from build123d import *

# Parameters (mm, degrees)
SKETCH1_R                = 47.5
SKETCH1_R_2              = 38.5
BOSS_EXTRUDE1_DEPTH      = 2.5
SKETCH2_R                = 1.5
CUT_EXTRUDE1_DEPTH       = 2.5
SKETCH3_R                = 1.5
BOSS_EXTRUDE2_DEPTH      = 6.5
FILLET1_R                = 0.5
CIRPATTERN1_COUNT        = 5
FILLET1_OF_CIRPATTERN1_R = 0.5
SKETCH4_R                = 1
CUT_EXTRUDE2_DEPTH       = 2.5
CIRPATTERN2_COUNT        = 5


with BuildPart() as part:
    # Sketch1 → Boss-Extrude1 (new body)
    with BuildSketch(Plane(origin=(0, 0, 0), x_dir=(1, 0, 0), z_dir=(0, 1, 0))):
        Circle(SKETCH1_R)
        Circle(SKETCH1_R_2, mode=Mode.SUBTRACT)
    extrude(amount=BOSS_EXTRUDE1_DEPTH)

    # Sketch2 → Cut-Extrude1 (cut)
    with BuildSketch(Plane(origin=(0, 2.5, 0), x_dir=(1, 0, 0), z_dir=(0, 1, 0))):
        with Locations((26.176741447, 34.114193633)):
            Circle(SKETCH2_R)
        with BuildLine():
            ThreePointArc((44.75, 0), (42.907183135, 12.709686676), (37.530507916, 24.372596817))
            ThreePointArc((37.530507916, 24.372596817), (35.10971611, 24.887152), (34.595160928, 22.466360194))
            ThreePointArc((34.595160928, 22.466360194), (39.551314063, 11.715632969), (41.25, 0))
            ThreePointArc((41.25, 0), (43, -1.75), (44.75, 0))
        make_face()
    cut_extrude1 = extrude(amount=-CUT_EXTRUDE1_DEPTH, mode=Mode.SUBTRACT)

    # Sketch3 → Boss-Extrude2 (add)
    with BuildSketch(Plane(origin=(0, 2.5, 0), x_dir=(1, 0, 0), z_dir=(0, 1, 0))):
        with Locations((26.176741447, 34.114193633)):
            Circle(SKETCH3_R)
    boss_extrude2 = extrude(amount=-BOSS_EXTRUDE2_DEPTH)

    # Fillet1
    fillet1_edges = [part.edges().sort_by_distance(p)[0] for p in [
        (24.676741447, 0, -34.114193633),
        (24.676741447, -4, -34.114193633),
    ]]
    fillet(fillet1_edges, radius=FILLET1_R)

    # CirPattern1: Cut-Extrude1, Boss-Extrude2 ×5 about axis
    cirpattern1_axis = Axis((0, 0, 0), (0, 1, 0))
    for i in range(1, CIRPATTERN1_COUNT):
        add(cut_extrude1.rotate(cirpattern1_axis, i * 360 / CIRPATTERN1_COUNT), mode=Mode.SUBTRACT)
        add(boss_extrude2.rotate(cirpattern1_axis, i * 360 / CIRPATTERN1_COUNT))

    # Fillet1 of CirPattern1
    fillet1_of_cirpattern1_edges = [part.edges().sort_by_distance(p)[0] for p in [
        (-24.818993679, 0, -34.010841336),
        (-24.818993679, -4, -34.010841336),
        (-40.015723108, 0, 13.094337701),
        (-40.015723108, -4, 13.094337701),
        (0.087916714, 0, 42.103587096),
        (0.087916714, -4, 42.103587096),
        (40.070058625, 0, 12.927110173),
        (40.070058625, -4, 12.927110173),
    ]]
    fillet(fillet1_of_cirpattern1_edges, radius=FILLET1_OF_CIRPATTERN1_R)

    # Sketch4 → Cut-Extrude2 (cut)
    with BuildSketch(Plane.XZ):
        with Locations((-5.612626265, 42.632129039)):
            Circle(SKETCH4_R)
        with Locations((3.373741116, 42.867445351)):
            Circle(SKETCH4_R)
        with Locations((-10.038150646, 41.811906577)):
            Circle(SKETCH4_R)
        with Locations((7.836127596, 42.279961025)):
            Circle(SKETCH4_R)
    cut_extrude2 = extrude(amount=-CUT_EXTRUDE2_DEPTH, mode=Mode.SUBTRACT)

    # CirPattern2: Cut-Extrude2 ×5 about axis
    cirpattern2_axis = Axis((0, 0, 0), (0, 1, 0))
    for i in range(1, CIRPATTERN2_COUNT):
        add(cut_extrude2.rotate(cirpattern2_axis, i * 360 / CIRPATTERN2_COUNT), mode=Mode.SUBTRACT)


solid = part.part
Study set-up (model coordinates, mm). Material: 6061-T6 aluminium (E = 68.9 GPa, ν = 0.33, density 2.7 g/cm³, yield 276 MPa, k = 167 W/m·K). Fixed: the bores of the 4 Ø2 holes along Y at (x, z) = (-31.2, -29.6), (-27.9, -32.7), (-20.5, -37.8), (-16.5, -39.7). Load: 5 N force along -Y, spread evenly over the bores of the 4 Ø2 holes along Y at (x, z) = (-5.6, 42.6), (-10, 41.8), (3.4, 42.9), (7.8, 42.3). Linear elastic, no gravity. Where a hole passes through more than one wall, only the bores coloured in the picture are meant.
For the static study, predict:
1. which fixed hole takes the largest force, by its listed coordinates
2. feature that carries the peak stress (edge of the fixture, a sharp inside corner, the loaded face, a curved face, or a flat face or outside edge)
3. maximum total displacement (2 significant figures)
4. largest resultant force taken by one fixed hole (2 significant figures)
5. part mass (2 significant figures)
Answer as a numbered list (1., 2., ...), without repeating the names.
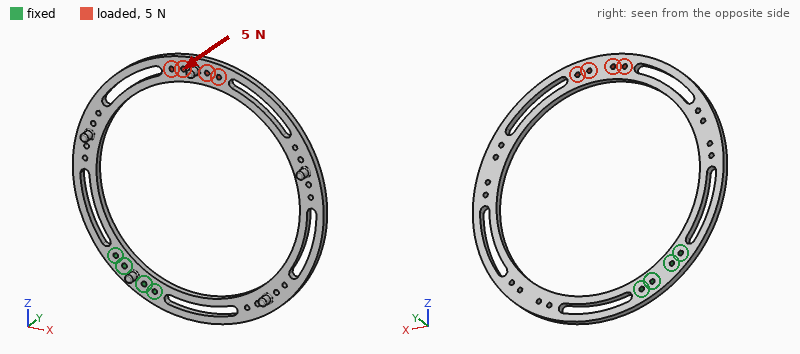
1. (-31.2, -29.6)
2. a flat face or outside edge
3. 1.4 mm
4. 13 N
5. 13 g
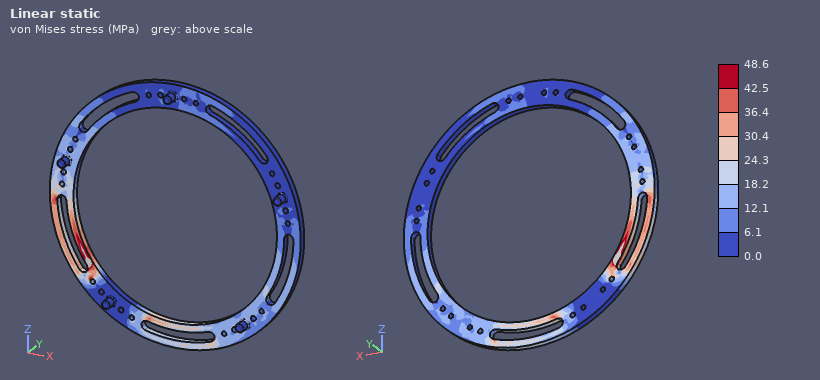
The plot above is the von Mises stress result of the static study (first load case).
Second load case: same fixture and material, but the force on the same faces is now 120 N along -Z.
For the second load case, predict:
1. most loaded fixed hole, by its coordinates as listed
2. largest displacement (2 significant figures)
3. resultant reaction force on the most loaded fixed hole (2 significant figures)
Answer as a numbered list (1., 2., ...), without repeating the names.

1. (-16.5, -39.7)
2. 0.78 mm
3. 280 N
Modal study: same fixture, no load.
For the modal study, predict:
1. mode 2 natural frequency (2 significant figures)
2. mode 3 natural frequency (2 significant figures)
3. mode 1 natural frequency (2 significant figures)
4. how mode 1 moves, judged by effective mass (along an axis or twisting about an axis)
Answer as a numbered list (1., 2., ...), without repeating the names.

1. 330 Hz
2. 520 Hz
3. 140 Hz
4. along Y
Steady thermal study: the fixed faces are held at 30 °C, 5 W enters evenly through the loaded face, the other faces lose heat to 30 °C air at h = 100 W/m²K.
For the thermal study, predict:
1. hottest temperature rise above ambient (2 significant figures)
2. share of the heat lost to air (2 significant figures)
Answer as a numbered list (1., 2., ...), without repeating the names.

1. 27 K
2. 93 %
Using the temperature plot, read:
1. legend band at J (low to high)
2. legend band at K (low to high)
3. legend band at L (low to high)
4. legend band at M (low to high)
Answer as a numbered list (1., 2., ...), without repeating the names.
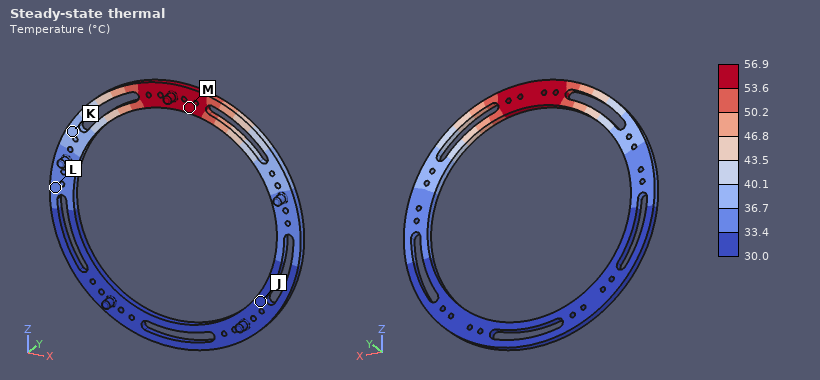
1. 30.0 to 33.4 °C
2. 36.7 to 40.1 °C
3. 33.4 to 36.7 °C
4. 53.6 to 56.9 °C
